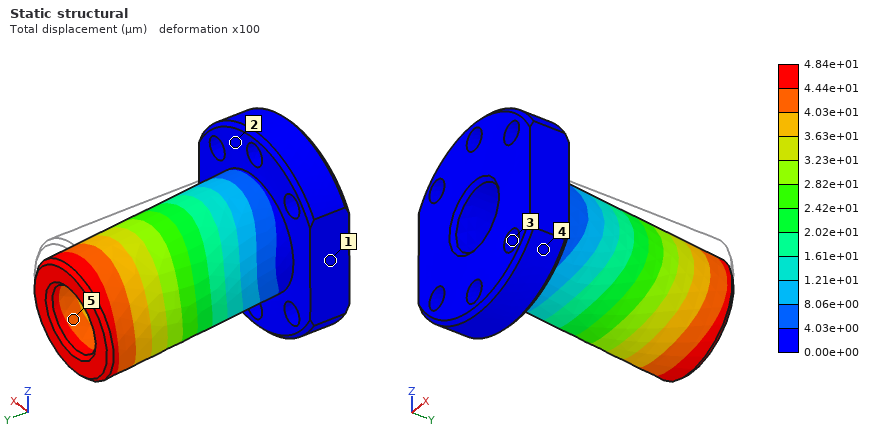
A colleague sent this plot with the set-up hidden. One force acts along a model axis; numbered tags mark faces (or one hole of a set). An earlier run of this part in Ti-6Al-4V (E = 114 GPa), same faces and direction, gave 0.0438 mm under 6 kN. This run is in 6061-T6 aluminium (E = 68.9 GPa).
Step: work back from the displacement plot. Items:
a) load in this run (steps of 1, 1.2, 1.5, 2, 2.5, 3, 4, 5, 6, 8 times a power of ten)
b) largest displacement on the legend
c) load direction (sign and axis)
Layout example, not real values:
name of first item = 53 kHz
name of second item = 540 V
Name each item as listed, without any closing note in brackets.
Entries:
load in this run = 4 kN
largest displacement on the legend = 4.84e+01 µm
load direction = -Z
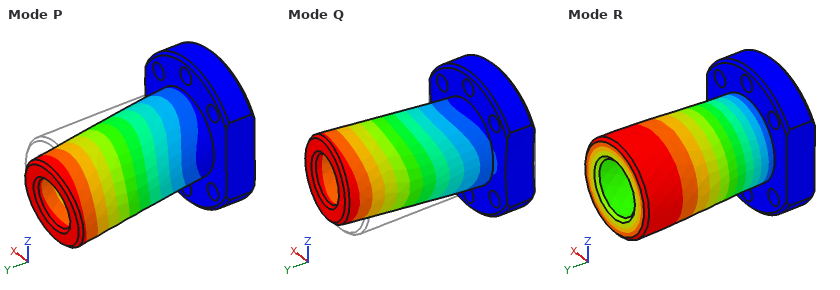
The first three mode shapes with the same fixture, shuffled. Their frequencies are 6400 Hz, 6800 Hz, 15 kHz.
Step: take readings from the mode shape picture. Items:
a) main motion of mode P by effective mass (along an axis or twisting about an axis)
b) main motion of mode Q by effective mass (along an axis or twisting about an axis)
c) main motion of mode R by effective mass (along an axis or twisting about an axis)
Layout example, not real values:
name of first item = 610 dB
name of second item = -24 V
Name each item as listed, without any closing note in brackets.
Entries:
main motion of mode P by effective mass = along Z
main motion of mode Q by effective mass = along X
main motion of mode R by effective mass = twisting about Y
